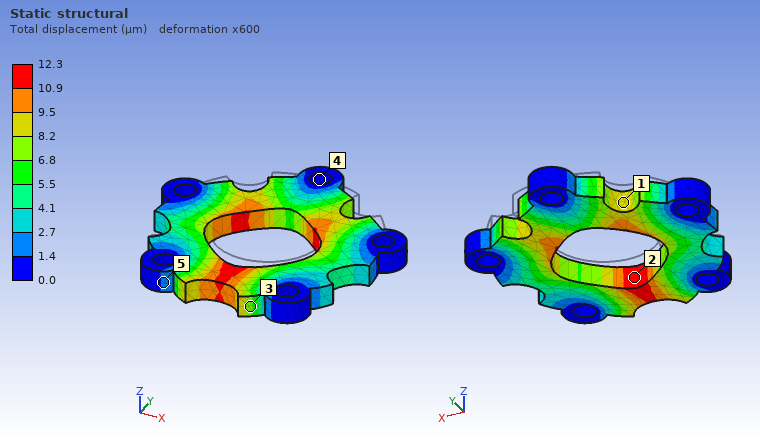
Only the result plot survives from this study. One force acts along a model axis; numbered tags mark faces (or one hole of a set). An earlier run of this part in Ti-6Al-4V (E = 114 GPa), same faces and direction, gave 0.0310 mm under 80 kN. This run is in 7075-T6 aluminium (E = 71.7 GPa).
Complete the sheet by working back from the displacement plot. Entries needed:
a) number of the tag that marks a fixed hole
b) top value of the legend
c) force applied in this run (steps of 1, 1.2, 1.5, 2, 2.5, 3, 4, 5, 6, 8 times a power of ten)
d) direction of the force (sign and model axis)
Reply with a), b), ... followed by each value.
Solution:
a) 4
b) 12.3 µm
c) 20 kN
d) -Y
